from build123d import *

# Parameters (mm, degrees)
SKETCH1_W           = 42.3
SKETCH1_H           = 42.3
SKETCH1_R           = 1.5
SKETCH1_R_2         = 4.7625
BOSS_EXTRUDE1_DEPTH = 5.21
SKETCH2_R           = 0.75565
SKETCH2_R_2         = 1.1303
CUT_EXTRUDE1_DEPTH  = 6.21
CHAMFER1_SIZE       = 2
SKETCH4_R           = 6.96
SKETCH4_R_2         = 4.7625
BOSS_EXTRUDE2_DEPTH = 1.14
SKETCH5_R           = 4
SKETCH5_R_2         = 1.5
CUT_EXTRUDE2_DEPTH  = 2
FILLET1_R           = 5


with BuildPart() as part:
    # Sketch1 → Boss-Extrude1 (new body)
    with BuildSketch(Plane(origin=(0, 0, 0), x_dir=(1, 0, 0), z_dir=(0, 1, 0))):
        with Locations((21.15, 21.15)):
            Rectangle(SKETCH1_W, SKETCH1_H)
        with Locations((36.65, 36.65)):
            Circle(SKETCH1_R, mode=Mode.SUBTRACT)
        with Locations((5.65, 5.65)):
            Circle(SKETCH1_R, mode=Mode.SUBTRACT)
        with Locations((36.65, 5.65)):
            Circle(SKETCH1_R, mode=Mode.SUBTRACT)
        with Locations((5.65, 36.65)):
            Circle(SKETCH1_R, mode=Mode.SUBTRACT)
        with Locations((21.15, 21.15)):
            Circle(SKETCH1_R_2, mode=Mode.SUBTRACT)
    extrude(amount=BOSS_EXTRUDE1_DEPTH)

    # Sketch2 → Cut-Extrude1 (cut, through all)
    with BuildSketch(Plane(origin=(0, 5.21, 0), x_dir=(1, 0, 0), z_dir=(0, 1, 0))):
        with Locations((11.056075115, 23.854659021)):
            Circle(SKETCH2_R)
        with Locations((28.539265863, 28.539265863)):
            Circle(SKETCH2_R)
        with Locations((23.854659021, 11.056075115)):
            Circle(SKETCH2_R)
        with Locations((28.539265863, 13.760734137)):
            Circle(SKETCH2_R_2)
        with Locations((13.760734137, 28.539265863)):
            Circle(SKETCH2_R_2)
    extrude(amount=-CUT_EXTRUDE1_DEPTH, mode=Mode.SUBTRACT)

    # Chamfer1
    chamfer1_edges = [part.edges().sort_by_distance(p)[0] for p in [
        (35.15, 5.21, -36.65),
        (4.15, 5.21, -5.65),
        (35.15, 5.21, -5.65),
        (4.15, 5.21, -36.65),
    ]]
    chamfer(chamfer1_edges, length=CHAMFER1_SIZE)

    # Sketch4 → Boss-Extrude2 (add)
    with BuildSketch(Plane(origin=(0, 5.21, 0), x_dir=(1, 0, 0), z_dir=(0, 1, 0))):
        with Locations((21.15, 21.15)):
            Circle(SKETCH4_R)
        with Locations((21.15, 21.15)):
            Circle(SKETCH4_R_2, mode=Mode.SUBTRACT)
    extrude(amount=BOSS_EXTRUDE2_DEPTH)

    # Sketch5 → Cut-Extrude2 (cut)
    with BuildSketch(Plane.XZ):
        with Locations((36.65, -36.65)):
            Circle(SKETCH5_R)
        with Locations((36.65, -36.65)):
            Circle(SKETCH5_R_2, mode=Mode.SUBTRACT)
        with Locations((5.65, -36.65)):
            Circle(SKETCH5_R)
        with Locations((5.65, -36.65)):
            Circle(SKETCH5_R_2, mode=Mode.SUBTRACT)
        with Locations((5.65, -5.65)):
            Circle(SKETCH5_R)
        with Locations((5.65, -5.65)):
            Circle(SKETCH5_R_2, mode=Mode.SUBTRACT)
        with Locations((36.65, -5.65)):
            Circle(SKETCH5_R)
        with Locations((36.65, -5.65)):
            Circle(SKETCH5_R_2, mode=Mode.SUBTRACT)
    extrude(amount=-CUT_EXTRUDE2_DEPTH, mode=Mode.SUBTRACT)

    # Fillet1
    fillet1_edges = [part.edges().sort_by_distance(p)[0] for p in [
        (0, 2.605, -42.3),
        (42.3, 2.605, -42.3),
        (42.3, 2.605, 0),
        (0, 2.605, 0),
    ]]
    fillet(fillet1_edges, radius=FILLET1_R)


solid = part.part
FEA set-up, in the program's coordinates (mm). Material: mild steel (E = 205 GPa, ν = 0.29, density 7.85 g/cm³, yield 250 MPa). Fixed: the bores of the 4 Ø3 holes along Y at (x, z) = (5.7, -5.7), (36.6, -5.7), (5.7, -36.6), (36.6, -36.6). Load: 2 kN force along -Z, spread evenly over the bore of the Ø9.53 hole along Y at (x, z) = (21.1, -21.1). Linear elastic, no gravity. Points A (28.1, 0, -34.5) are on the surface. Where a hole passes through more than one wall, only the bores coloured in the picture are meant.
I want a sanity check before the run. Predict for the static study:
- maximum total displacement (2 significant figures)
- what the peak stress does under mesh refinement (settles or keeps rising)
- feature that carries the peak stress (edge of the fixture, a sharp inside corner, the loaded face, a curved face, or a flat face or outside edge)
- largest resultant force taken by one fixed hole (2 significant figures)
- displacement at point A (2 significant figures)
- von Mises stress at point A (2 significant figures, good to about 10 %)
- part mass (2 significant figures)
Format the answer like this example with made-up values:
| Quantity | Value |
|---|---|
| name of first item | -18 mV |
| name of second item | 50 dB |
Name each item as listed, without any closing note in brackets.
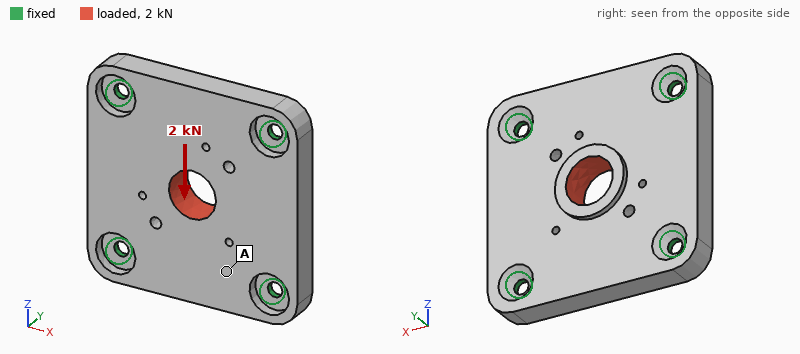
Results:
| Quantity | Value |
|---|---|
| maximum total displacement | 1.9 µm |
| what the peak stress does under mesh refinement | keeps rising |
| feature that carries the peak stress | edge of the fixture |
| largest resultant force taken by one fixed hole | 530 N |
| displacement at point A | 1.1 µm |
| von Mises stress at point A | 8.9 MPa |
| part mass | 65 g |
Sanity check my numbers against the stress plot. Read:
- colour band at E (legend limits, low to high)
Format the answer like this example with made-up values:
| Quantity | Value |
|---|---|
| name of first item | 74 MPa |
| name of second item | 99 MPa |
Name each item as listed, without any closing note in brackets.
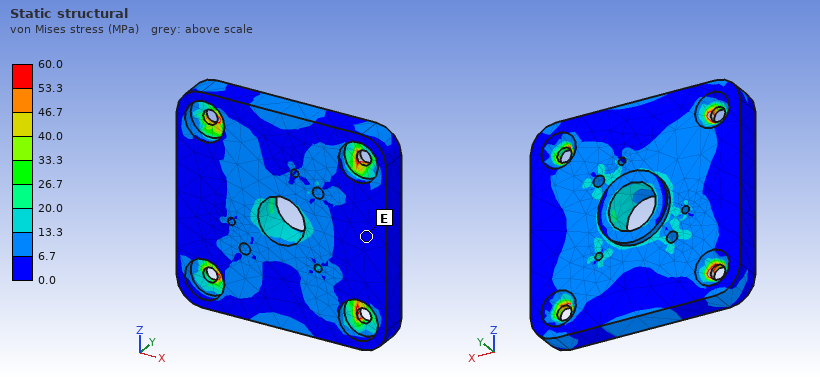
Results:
| Quantity | Value |
|---|---|
| colour band at E | 0.0 to 6.7 MPa |
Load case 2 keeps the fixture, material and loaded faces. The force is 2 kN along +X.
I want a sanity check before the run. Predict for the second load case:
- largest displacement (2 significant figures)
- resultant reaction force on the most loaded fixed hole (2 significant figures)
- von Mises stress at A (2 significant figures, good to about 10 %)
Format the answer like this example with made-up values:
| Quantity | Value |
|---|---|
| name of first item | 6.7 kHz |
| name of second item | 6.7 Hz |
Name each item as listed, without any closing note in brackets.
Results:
| Quantity | Value |
|---|---|
| largest displacement | 1.9 µm |
| resultant reaction force on the most loaded fixed hole | 530 N |
| von Mises stress at A | 6.1 MPa |
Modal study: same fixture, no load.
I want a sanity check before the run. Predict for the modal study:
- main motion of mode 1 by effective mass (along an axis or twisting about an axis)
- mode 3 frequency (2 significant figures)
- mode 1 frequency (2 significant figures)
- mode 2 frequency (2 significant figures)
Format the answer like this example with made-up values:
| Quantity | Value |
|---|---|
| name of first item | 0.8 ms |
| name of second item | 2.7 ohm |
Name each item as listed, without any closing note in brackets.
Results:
| Quantity | Value |
|---|---|
| main motion of mode 1 by effective mass | along Y |
| mode 3 frequency | 17 kHz |
| mode 1 frequency | 12 kHz |
| mode 2 frequency | 16 kHz |
